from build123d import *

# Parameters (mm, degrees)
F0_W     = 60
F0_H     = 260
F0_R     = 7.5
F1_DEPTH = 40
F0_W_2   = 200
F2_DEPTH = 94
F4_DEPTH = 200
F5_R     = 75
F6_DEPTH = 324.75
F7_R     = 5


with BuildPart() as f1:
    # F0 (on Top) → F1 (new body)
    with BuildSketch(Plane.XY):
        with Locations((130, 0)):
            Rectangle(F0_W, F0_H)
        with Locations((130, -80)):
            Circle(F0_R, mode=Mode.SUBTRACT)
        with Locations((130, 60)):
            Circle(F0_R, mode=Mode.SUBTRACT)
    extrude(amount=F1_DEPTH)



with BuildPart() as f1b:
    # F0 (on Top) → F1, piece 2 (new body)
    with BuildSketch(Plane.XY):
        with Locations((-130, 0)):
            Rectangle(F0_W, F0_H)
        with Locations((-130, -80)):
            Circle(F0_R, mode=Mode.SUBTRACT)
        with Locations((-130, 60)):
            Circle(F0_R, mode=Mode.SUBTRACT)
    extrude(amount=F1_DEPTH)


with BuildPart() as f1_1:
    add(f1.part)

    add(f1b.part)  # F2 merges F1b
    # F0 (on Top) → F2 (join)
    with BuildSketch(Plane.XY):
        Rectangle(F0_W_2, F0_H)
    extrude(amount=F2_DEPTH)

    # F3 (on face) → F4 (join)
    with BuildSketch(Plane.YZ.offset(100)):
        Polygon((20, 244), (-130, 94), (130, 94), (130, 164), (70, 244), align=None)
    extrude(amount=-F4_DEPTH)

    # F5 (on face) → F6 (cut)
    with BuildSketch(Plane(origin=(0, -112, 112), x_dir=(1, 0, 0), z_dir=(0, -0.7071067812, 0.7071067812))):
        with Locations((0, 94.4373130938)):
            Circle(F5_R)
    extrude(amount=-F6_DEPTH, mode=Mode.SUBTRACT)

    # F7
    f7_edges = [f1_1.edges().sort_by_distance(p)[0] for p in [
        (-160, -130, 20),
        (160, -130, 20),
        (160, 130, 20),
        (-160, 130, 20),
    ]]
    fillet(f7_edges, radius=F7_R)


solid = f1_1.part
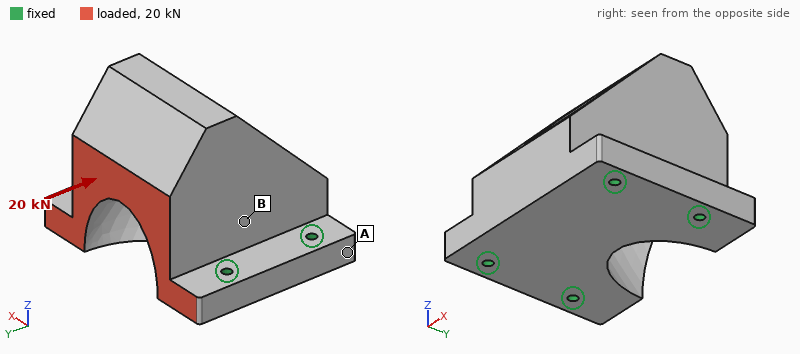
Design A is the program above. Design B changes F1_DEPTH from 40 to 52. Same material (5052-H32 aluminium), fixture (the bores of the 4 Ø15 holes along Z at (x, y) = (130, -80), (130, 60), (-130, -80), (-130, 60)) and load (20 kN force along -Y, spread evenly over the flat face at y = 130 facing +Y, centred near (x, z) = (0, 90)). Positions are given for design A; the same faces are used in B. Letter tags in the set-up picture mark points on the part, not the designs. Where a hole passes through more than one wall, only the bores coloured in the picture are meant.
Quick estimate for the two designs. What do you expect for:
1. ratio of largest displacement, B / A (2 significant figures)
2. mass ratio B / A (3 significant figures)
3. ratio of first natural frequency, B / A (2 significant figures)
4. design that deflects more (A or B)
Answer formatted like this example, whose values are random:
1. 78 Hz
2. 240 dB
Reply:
1. 0.66
2. 1.05
3. 1.2
4. A
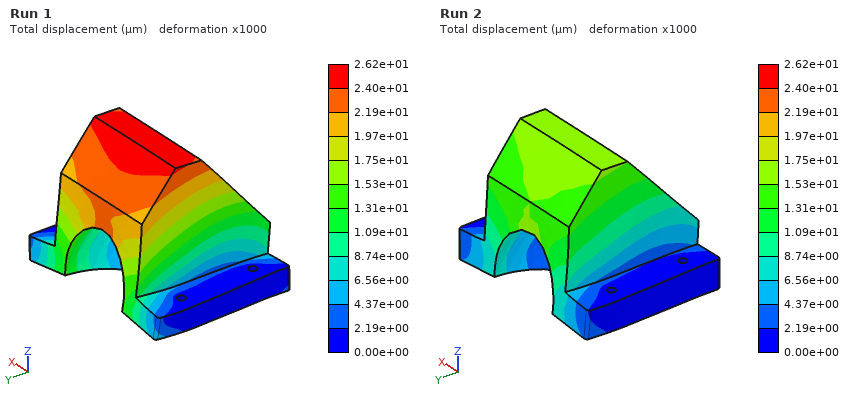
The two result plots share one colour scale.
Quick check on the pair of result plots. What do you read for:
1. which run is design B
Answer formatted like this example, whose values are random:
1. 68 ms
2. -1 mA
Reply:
1. Run 2
